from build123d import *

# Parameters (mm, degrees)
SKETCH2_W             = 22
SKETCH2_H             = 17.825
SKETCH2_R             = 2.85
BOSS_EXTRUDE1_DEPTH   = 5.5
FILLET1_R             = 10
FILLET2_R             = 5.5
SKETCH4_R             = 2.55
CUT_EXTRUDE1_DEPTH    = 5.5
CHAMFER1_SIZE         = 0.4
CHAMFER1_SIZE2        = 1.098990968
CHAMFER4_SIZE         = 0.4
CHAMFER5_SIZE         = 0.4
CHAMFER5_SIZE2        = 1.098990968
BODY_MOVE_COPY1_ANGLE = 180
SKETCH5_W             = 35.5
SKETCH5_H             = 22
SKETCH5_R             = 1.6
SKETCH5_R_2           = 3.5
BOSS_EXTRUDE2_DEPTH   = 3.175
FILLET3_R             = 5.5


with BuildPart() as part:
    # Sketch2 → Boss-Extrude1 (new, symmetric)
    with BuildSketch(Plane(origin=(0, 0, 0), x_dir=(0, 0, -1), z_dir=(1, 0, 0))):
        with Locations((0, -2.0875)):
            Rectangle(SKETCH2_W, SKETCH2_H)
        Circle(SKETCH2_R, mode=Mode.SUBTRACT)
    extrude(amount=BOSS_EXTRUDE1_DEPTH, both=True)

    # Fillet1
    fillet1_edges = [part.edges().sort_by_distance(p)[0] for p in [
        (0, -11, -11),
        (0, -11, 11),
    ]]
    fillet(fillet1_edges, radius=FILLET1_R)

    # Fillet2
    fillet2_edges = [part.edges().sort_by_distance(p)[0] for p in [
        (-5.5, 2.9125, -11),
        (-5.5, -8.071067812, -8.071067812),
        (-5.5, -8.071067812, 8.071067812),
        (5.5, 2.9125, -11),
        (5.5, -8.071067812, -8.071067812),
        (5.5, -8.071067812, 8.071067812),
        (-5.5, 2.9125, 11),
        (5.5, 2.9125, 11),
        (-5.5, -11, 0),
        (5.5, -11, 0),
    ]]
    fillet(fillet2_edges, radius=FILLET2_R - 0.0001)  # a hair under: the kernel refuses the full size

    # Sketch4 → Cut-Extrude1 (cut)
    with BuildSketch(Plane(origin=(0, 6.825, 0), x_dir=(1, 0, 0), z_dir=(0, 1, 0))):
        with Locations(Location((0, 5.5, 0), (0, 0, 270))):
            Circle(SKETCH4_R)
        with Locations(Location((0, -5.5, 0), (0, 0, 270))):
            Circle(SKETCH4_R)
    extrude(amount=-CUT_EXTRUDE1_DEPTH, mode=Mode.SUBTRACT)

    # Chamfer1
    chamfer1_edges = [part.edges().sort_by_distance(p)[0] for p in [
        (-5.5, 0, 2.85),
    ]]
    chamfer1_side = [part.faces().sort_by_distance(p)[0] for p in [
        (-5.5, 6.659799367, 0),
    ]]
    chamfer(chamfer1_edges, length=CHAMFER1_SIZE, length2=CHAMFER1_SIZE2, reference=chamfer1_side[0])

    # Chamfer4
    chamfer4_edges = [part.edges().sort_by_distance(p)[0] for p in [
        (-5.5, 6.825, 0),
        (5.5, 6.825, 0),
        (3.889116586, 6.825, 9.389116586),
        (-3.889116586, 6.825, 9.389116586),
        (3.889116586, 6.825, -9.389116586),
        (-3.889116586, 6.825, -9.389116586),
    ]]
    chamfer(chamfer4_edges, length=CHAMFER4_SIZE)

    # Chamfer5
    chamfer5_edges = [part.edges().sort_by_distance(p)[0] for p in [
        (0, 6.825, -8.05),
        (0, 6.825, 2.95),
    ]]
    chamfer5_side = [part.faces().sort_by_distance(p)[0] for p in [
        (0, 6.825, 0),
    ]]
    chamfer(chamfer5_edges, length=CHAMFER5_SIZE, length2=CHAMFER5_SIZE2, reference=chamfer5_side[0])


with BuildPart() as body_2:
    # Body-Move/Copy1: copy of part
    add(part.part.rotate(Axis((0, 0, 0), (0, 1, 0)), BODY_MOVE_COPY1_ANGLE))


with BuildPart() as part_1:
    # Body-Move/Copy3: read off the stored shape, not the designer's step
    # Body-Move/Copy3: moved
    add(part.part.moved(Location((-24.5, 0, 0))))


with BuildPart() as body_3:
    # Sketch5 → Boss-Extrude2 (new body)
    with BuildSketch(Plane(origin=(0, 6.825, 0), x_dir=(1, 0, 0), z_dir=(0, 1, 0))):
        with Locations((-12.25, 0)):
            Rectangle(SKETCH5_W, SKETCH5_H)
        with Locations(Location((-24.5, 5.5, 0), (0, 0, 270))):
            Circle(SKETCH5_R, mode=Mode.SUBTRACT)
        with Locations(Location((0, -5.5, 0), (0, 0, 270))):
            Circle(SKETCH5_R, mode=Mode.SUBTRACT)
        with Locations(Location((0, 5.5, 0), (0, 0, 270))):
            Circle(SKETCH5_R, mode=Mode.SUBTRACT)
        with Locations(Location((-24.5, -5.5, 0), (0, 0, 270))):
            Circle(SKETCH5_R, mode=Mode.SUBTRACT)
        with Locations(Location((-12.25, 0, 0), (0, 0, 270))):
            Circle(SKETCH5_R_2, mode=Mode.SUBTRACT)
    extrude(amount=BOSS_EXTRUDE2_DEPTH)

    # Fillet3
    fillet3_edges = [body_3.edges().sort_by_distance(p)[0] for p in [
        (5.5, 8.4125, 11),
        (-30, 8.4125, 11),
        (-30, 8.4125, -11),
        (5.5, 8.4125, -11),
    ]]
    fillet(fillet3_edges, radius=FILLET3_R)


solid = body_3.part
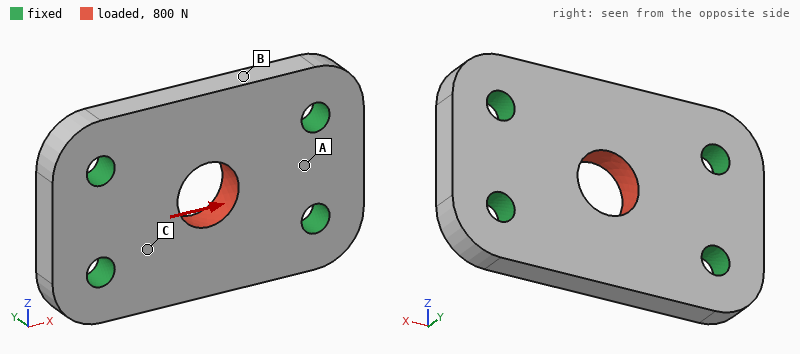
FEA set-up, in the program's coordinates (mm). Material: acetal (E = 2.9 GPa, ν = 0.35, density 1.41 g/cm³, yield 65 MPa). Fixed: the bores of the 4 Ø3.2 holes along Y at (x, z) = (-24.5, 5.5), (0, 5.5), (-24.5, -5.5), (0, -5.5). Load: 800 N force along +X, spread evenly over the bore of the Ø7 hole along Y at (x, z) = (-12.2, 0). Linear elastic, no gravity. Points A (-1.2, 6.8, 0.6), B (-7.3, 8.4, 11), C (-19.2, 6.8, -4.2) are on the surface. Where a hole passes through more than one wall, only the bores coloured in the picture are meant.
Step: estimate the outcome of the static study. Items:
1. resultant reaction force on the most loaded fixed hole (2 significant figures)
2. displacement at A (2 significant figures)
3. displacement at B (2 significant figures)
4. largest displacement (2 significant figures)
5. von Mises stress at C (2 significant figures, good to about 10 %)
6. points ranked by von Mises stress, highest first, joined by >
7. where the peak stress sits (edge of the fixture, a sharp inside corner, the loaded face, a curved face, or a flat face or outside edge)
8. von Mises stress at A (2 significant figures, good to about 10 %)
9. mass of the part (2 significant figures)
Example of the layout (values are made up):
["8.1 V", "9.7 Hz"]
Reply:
["210 N", "9.8 µm", "11 µm", "35 µm", "9.5 MPa", "C > A > B", "the loaded face", "3.8 MPa", "3.1 g"]
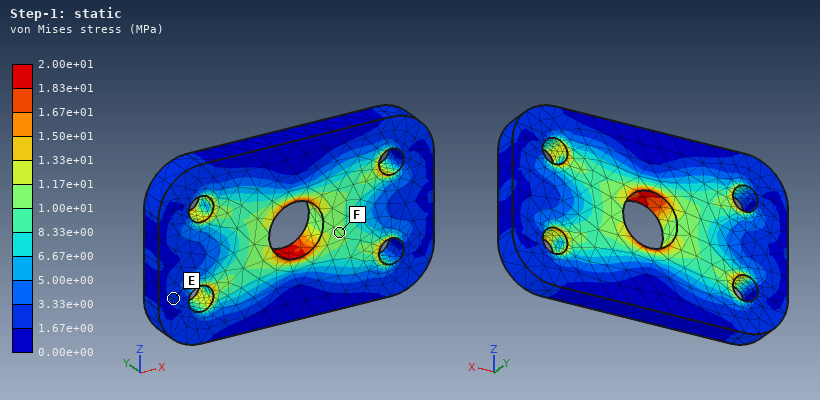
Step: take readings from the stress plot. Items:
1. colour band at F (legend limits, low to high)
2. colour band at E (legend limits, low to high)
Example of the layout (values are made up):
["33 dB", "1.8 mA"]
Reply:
["1.00e+01 to 1.17e+01 MPa", "1.67e+00 to 3.33e+00 MPa"]
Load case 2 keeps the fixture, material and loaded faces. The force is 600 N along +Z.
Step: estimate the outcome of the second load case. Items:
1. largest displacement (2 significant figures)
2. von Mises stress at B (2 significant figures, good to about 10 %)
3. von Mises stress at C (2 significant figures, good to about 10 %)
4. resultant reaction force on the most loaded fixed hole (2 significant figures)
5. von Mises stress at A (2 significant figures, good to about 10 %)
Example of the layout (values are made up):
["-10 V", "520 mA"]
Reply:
["59 µm", "5.3 MPa", "9.0 MPa", "180 N", "5.9 MPa"]
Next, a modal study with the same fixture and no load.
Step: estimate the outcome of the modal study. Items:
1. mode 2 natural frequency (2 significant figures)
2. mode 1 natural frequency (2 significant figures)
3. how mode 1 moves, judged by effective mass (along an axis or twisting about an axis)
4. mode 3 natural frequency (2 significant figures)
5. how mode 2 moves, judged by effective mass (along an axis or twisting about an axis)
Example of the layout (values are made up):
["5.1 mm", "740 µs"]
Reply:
["8500 Hz", "7800 Hz", "along Y", "14 kHz", "twisting about X"]
